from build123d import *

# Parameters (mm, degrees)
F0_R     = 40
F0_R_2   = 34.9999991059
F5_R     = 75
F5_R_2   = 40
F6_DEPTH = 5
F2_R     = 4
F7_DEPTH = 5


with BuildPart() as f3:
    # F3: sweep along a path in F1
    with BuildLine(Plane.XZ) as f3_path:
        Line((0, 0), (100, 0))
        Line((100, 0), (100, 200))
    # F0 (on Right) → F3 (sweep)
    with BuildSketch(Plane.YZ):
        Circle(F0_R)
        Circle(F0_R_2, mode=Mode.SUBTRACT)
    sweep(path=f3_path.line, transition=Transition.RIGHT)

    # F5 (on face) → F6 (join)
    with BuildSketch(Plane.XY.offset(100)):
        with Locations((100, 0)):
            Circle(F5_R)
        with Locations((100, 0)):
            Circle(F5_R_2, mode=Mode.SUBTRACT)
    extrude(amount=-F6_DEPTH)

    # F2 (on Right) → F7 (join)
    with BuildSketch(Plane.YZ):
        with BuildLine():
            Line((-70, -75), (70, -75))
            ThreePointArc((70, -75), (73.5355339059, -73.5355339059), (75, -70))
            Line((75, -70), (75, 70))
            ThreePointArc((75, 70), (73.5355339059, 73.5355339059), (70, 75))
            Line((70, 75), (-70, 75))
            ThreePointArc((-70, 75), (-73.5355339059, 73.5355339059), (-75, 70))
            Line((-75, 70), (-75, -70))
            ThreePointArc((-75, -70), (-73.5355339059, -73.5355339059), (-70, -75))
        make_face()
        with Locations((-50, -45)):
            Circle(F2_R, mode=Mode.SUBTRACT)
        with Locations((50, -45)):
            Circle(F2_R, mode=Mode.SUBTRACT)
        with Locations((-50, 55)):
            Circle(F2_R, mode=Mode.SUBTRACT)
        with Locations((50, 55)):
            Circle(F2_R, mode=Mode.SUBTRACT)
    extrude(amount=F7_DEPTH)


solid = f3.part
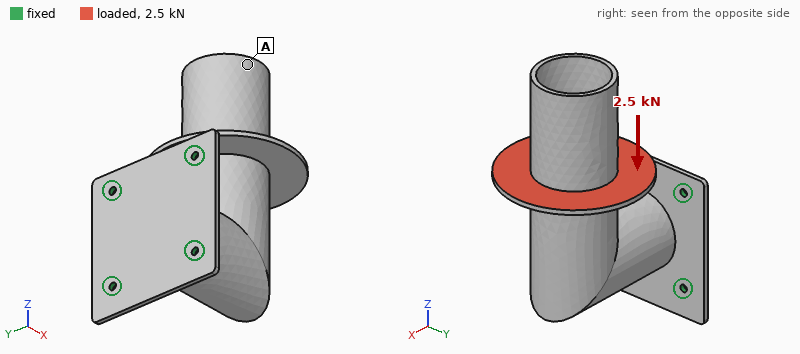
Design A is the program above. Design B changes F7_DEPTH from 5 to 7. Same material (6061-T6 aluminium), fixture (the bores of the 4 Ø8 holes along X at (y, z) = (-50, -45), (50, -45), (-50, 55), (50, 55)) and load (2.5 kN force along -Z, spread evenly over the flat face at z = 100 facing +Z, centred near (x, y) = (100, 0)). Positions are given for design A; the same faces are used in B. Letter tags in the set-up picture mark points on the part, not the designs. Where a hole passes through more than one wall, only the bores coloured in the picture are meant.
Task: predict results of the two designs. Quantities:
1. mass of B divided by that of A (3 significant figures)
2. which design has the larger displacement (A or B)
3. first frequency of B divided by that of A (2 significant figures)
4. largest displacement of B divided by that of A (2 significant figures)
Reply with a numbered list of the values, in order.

1. 1.08
2. A
3. 1.4
4. 0.48
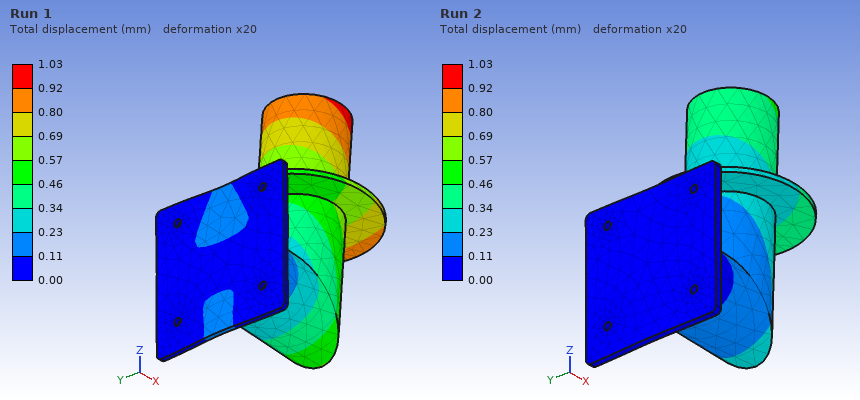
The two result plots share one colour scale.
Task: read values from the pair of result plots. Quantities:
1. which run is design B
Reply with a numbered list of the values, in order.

1. Run 2
